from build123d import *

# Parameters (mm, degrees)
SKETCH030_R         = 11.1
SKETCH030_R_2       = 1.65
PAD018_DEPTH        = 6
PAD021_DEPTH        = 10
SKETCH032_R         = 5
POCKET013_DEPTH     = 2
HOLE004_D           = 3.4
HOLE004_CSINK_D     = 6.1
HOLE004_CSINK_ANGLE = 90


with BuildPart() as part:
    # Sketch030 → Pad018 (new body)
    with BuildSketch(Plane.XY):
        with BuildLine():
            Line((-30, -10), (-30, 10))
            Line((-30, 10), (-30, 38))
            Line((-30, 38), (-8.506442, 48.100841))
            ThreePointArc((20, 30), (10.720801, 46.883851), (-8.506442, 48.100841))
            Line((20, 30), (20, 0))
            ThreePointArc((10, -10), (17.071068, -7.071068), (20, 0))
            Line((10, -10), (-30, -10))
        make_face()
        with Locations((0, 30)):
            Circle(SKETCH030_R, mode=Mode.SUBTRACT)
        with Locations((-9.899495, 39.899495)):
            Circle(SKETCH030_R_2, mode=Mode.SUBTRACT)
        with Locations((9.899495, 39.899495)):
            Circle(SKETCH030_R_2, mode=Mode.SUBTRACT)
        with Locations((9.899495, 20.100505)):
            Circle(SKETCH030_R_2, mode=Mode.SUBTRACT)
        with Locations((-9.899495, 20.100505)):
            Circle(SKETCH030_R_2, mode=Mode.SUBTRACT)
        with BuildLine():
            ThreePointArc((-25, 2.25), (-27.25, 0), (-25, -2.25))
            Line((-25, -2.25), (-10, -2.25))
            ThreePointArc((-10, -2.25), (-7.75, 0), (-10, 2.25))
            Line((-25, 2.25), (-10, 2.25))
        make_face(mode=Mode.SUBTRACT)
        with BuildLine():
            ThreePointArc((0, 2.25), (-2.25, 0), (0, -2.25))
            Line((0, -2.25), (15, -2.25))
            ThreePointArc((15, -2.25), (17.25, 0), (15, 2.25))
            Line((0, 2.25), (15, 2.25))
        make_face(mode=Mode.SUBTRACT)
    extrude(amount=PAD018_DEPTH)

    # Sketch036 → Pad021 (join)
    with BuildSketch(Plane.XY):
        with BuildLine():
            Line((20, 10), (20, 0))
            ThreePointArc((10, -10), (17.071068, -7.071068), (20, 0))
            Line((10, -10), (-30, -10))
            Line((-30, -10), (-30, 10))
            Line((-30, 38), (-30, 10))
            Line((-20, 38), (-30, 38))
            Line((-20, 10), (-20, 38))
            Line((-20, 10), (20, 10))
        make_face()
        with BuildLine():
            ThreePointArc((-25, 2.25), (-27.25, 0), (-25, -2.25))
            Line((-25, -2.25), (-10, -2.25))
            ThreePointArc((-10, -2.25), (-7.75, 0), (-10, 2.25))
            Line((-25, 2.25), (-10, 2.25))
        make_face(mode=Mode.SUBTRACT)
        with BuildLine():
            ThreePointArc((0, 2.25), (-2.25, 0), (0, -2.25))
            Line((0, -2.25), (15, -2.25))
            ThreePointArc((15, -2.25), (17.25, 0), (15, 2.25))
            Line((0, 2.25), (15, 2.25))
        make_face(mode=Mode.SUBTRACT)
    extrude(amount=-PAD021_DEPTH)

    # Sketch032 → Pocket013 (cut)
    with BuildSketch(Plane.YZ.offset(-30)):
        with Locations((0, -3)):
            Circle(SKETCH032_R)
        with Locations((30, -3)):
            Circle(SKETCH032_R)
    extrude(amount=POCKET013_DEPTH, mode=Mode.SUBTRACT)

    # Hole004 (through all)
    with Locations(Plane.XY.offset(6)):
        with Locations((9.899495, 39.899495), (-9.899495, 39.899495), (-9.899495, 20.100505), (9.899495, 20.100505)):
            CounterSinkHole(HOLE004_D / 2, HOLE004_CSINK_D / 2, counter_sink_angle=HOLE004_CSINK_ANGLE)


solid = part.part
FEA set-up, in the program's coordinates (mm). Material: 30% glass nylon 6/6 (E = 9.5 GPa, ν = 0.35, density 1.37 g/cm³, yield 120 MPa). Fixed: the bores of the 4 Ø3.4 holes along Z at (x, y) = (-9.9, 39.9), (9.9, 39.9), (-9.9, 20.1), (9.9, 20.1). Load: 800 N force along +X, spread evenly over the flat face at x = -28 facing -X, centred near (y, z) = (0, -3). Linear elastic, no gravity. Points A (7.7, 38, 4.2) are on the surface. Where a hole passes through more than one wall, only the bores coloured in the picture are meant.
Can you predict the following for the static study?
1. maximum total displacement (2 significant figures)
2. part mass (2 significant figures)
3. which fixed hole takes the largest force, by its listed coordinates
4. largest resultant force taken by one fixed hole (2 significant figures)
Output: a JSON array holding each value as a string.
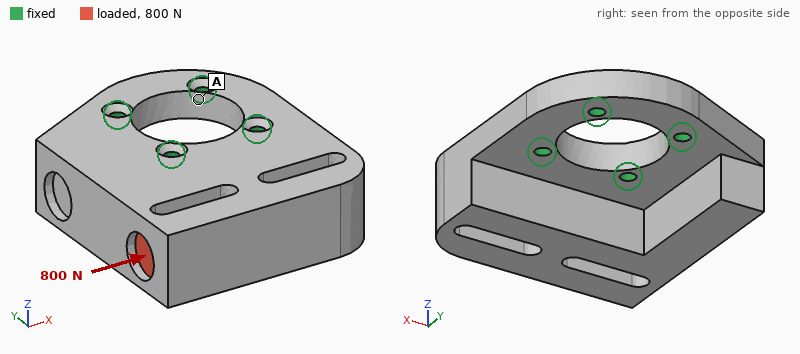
["0.10 mm", "32 g", "(-9.9, 20.1)", "730 N"]
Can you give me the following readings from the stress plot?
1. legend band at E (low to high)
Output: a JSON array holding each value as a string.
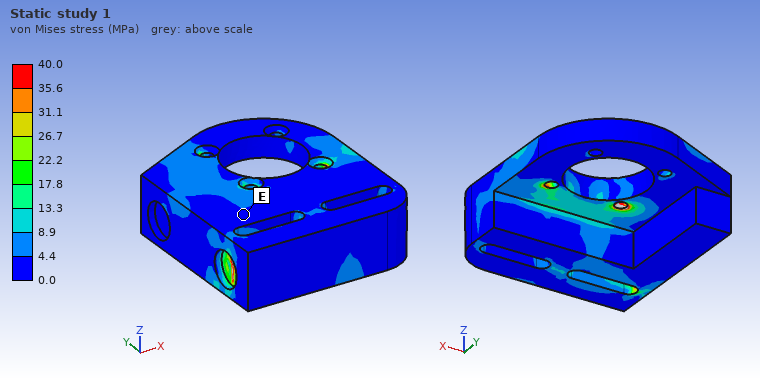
["0.0 to 4.4 MPa"]
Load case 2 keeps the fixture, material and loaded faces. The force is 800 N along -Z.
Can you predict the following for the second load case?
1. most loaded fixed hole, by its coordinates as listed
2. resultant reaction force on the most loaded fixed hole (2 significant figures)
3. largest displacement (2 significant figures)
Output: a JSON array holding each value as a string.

["(-9.9, 20.1)", "1.6 kN", "0.80 mm"]
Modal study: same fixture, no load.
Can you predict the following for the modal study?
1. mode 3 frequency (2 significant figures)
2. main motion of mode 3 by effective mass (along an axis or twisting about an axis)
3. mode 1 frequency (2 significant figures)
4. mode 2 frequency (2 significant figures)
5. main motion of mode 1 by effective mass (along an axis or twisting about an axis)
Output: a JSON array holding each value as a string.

["5000 Hz", "along X", "1800 Hz", "2900 Hz", "along Z"]
